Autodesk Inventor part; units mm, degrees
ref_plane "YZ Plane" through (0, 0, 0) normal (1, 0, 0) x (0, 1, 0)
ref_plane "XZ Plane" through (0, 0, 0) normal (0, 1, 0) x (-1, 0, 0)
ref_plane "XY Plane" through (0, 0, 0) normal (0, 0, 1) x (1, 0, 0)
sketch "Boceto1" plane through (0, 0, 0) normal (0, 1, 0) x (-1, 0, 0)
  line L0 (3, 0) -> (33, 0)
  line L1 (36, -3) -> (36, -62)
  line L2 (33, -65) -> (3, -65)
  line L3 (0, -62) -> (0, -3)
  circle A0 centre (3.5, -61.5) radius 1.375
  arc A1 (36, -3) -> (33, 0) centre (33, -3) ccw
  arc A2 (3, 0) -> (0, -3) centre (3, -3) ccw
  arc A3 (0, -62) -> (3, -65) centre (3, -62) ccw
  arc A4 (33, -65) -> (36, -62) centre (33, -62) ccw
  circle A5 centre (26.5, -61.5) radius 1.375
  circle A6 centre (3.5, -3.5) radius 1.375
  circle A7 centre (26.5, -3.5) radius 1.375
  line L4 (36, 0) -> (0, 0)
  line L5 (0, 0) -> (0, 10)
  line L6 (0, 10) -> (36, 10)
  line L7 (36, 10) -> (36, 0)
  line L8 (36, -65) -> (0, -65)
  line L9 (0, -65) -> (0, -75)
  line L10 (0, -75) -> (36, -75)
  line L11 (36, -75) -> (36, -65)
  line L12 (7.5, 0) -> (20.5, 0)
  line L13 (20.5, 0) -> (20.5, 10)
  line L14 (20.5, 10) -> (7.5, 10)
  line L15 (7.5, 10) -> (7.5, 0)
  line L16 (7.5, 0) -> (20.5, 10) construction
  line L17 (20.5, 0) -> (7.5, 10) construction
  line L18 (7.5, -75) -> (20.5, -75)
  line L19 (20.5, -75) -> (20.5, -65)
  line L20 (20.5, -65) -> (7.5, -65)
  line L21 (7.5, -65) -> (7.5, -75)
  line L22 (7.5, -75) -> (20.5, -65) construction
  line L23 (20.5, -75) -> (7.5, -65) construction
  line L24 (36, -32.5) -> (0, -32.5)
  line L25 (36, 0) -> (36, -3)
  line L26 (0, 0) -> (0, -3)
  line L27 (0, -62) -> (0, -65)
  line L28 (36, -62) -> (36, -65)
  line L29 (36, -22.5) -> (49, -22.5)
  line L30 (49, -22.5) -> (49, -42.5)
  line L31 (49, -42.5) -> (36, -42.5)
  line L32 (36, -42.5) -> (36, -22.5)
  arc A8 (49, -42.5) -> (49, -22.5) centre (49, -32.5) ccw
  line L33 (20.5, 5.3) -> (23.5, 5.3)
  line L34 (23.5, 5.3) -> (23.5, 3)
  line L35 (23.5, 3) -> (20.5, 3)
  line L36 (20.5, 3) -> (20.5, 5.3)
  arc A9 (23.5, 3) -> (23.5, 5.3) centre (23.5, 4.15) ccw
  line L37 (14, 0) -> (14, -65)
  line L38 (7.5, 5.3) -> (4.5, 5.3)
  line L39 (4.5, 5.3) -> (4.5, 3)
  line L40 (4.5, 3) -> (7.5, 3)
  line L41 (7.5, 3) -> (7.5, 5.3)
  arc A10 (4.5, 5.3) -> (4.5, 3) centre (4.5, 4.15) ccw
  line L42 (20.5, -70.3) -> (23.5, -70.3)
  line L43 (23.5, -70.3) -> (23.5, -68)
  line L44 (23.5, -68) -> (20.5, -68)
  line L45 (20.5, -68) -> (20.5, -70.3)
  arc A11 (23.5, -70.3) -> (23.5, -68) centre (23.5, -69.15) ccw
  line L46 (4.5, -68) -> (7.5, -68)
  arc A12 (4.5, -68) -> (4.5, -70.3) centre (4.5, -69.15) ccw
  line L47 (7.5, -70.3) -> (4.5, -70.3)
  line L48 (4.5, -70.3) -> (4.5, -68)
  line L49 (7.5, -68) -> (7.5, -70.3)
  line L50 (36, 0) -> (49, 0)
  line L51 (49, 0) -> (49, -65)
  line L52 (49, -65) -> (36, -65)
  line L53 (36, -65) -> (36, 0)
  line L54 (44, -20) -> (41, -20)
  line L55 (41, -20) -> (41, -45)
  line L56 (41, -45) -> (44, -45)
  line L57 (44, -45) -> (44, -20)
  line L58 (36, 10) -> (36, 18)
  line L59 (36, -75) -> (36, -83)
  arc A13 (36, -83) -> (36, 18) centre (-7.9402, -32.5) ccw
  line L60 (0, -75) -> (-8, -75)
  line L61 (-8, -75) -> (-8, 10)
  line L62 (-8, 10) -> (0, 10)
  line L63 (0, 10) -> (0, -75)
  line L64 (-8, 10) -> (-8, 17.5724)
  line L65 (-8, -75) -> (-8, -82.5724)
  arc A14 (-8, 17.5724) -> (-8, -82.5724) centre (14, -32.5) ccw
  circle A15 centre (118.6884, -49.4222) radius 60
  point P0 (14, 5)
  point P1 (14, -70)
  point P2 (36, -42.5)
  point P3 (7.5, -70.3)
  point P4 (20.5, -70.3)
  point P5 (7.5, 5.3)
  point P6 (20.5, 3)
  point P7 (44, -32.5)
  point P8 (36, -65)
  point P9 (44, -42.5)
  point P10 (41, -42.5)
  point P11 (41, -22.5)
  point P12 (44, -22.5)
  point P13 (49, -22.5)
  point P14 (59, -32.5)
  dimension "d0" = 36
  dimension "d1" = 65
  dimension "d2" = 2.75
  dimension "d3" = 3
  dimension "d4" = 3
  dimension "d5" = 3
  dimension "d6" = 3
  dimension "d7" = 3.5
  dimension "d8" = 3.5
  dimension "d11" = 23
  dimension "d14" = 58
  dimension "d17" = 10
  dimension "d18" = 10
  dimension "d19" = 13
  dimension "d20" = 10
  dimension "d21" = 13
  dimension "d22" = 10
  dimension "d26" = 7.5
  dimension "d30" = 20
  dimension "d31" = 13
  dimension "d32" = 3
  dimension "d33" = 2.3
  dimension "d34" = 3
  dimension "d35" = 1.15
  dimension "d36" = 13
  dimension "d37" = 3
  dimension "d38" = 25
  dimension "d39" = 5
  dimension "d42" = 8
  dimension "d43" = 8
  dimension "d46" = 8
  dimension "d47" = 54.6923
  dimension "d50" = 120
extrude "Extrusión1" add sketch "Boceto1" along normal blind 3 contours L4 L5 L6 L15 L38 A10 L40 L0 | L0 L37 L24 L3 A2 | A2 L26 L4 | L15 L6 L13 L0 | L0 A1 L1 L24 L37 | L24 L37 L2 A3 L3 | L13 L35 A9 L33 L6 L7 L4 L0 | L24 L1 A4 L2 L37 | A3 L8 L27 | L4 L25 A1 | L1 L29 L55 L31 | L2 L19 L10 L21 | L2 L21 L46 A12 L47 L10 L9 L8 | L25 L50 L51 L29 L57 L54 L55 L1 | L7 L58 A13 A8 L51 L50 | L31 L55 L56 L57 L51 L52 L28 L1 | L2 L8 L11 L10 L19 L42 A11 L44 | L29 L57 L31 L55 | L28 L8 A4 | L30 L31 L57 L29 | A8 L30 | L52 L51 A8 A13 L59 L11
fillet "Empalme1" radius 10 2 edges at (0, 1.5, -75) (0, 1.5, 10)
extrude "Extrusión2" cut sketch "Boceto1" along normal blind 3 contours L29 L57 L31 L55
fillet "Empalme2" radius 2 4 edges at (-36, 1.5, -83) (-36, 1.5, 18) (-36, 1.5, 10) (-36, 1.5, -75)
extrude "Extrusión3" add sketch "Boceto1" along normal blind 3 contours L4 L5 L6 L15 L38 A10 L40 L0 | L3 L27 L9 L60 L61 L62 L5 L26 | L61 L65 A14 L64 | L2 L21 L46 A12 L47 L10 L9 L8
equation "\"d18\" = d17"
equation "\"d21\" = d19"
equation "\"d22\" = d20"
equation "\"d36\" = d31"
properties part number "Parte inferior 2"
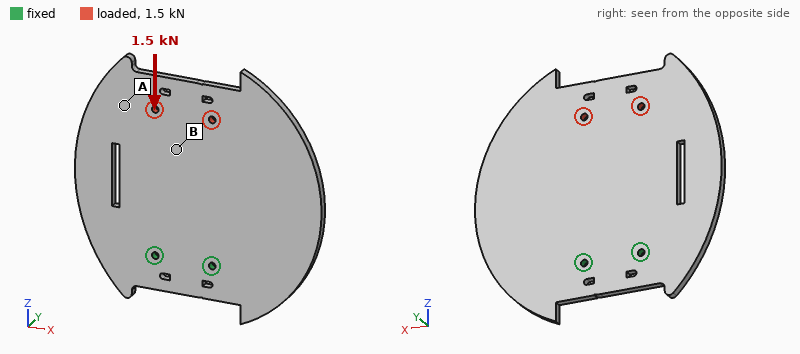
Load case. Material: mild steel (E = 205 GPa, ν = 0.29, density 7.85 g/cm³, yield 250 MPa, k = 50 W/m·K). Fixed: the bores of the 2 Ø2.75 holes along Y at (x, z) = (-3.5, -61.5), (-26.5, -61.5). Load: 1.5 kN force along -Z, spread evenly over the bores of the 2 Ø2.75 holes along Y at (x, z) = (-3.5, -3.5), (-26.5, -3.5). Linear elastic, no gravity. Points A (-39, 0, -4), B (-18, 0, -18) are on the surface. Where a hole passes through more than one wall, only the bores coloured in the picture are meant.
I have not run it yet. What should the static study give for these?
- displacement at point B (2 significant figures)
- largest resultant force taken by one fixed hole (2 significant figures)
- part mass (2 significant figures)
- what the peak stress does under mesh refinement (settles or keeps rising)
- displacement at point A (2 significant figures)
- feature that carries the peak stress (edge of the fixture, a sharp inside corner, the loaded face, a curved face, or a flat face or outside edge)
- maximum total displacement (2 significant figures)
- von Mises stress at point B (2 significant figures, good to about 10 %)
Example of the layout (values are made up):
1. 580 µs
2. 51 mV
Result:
1. 2.6 µm
2. 750 N
3. 180 g
4. keeps rising
5. 2.5 µm
6. edge of the fixture
7. 3.8 µm
8. 10 MPa
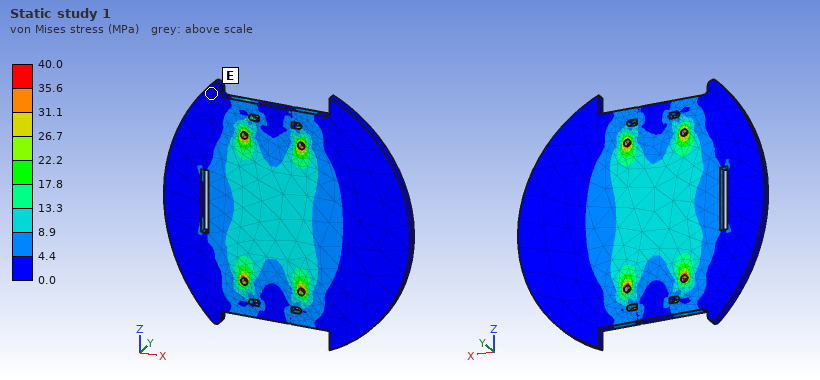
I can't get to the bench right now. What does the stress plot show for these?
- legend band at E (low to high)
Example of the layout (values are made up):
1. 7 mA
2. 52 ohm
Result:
1. 0.0 to 4.4 MPa
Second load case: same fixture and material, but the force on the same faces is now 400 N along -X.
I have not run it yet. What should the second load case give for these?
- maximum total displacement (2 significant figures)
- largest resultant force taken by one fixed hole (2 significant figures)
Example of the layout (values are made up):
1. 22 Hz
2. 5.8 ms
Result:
1. 13 µm
2. 970 N
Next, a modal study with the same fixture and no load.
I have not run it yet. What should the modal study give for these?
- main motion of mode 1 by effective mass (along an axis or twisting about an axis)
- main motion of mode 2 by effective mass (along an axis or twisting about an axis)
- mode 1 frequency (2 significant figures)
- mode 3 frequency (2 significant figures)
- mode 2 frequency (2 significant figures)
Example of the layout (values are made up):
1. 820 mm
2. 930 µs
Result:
1. along Y
2. twisting about Z
3. 420 Hz
4. 1600 Hz
5. 760 Hz
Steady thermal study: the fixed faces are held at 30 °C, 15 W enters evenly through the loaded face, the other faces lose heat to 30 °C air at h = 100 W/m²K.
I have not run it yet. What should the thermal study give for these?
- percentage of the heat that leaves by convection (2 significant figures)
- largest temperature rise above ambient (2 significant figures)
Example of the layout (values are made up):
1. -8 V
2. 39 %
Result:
1. 91 %
2. 37 K
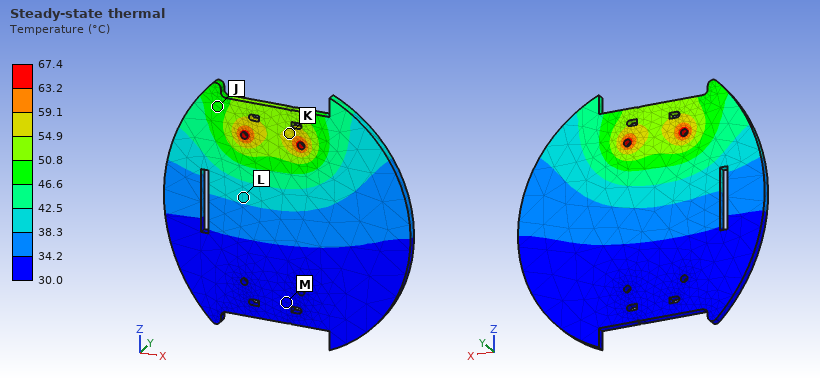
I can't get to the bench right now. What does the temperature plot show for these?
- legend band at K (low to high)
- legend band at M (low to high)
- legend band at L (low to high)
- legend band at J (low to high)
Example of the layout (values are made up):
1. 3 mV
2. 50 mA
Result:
1. 54.9 to 59.1 °C
2. 30.0 to 34.2 °C
3. 38.3 to 42.5 °C
4. 46.6 to 50.8 °C
